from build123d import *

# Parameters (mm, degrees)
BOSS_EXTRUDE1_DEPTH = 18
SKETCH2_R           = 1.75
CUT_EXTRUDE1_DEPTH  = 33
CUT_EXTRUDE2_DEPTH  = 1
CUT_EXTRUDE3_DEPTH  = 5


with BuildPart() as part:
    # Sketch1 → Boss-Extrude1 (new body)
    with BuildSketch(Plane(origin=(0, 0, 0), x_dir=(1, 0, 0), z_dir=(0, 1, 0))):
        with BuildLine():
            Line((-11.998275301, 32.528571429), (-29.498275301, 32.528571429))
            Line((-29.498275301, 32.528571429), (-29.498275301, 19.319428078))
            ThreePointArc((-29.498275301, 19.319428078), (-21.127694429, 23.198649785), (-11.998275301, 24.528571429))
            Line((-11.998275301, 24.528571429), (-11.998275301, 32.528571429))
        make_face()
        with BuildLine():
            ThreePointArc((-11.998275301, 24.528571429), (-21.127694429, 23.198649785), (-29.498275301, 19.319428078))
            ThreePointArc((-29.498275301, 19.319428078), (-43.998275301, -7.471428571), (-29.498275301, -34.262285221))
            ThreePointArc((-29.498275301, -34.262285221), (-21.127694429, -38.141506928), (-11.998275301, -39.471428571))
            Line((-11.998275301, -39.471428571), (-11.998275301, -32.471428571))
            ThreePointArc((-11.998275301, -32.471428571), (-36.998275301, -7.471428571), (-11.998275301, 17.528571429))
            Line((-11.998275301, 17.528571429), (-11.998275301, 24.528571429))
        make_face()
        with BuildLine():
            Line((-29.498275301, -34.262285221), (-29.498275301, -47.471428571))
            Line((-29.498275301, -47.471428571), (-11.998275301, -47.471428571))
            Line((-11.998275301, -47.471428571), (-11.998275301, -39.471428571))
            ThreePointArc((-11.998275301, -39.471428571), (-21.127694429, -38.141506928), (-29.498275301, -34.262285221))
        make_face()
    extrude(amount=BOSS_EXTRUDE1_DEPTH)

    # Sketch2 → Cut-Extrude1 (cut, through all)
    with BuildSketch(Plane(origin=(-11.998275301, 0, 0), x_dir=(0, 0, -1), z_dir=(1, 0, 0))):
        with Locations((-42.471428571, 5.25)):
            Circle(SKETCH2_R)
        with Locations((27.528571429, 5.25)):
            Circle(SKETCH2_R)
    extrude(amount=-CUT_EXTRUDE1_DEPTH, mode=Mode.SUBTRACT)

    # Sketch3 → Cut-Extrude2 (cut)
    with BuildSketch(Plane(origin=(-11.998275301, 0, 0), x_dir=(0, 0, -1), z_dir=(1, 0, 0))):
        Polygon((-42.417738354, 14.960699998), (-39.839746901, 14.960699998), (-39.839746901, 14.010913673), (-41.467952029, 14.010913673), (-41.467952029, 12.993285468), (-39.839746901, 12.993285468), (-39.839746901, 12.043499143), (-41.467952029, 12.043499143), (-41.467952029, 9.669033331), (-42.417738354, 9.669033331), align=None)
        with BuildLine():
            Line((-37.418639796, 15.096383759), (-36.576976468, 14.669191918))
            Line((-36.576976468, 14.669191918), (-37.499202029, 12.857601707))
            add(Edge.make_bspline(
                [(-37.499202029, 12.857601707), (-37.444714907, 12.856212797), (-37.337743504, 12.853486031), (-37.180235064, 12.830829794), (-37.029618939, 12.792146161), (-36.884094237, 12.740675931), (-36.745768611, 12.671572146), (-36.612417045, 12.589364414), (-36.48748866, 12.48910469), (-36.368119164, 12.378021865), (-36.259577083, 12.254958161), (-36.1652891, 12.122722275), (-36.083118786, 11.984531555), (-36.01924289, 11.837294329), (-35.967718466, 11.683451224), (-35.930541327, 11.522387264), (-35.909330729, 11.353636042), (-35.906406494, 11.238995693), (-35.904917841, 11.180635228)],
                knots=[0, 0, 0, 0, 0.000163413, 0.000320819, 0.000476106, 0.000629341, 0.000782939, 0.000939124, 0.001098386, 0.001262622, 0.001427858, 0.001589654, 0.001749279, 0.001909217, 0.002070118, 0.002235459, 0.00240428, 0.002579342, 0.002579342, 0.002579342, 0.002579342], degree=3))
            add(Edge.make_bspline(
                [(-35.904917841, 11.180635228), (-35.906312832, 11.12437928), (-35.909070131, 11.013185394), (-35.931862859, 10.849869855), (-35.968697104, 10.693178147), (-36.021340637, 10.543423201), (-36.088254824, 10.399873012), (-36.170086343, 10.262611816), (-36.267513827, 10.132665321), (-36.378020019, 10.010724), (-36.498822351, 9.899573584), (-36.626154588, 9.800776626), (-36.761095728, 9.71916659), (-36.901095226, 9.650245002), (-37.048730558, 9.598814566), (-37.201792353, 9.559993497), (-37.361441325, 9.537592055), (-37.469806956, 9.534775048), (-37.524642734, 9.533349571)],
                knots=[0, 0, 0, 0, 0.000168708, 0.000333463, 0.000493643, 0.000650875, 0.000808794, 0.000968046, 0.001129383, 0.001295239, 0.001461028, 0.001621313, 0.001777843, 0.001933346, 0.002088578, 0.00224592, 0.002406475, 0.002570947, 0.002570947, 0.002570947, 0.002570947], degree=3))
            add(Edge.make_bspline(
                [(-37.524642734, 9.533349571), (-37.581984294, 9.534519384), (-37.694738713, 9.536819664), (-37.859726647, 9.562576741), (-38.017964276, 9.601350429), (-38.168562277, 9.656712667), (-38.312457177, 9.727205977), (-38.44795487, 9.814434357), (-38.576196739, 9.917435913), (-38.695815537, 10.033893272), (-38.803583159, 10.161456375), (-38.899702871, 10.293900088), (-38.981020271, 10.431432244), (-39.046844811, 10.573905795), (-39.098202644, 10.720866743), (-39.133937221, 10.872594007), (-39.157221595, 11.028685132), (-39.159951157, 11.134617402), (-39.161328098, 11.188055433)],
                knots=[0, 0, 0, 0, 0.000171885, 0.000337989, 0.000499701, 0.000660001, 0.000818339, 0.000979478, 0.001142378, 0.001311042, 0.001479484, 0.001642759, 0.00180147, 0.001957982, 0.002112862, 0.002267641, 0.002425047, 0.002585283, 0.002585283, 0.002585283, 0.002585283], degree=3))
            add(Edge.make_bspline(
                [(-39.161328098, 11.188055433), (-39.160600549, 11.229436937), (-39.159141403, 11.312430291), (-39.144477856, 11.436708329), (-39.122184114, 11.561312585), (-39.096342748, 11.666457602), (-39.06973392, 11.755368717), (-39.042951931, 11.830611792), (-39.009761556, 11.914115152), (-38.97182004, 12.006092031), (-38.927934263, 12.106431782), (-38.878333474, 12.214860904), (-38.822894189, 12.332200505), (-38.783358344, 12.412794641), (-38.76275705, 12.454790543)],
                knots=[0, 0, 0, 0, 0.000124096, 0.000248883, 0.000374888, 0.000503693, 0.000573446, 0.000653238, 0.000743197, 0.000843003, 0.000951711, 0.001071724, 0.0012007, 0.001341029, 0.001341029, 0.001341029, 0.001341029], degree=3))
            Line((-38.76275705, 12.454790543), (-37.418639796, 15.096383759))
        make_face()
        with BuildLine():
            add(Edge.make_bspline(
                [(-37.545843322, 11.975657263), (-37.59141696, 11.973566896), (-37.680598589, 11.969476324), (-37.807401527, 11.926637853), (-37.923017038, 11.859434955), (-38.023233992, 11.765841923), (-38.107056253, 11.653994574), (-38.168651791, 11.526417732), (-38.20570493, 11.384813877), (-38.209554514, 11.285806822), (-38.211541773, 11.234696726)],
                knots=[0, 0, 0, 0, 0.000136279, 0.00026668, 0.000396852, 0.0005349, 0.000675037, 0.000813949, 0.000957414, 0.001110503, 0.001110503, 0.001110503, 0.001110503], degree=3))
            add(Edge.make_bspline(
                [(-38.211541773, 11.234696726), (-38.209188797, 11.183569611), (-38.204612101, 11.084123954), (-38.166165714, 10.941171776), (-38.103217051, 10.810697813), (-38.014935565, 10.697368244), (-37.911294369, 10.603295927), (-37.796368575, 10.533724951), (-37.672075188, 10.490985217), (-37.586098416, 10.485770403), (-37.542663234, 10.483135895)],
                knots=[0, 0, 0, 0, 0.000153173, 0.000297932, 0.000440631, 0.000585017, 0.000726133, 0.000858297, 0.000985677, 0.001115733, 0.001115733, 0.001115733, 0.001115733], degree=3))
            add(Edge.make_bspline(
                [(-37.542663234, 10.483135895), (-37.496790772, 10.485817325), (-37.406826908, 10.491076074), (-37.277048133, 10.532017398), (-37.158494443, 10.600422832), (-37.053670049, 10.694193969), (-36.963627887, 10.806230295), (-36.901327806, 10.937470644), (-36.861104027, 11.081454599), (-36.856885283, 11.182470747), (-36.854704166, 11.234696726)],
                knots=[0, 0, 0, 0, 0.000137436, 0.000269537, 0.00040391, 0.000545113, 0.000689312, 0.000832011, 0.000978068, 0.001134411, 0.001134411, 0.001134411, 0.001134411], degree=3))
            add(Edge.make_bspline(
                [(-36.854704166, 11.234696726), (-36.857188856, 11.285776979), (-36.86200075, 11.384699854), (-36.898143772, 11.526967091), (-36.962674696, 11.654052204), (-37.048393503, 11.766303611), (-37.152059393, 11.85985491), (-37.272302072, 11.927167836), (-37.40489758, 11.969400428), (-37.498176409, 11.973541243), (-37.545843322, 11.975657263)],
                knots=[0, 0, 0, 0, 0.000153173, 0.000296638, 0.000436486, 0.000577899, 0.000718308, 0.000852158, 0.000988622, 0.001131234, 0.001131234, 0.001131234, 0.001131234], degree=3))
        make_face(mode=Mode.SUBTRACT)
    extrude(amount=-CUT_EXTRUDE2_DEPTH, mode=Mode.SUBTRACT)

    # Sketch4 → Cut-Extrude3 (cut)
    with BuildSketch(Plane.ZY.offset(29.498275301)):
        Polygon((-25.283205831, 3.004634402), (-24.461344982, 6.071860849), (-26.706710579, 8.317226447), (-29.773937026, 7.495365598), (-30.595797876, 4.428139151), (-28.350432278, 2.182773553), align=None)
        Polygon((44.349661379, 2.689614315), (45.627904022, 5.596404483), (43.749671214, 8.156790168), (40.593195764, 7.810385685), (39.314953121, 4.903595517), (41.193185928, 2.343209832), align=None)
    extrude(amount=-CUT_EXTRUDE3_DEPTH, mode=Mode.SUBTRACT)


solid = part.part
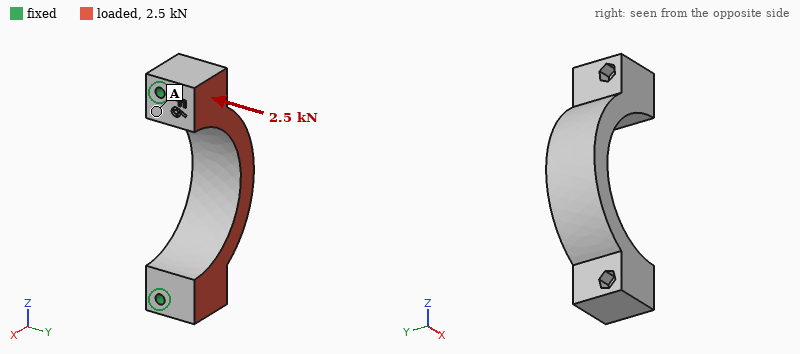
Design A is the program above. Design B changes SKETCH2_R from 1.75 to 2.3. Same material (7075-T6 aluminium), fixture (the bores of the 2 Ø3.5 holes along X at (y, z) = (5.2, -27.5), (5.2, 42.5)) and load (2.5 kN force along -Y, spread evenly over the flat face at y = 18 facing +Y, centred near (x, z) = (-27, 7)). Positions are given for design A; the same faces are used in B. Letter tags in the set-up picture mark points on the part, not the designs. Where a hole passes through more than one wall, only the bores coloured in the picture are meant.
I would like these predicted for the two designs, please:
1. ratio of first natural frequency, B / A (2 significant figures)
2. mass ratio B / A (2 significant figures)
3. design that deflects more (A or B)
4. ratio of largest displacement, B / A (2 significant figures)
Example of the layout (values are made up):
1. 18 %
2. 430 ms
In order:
1. 1.1
2. 0.99
3. A
4. 0.81
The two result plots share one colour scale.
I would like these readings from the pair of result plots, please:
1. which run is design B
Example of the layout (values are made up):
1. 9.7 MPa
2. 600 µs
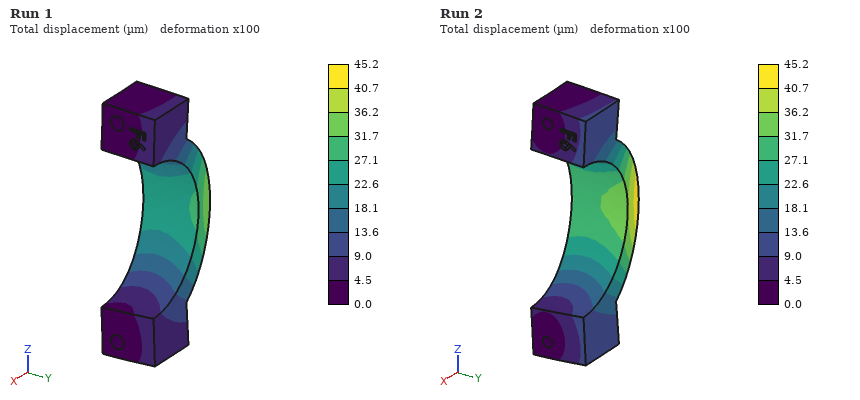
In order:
1. Run 1
